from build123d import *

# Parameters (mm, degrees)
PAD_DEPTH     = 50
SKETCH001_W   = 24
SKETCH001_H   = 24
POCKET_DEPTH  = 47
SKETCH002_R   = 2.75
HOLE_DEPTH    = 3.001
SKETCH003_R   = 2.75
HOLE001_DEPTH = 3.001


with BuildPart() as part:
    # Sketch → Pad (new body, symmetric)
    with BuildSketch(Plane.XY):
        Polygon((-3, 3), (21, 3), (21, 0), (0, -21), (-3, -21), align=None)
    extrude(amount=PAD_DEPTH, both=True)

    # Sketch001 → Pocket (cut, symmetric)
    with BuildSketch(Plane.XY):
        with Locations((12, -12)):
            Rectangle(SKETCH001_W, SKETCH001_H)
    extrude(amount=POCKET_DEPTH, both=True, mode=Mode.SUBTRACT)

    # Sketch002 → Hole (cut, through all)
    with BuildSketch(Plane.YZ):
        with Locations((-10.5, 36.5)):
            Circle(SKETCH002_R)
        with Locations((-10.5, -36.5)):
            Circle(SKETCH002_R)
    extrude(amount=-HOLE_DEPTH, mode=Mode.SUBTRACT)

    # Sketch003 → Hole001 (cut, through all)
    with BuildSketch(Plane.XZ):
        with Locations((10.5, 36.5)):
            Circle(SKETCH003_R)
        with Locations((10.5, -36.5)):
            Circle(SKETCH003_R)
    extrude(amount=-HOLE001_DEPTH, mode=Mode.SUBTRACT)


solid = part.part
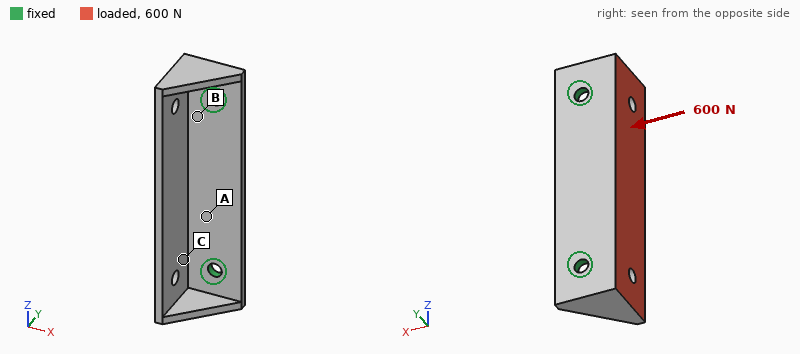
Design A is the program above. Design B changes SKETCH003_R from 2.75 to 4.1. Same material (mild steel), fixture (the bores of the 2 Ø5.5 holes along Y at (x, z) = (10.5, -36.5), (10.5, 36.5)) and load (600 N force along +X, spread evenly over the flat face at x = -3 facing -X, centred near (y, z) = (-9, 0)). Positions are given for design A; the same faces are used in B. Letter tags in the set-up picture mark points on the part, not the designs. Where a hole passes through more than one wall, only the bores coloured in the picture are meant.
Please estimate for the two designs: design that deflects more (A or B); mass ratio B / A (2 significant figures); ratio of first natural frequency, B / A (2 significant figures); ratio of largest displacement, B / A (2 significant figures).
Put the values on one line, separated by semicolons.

A; 0.99; 1.1; 0.86
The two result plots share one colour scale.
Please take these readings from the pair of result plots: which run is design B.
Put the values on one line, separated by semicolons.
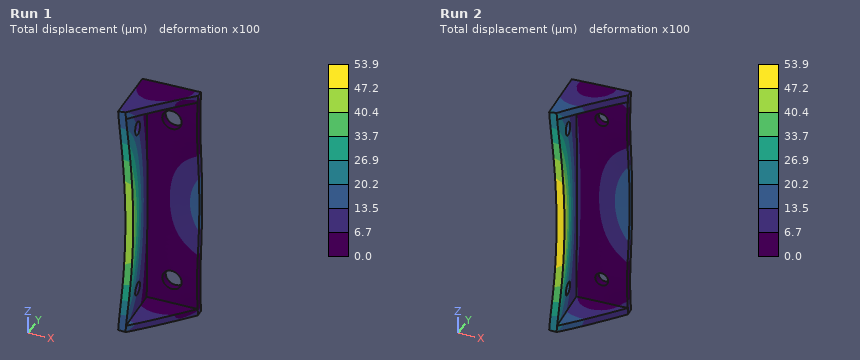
Run 1
